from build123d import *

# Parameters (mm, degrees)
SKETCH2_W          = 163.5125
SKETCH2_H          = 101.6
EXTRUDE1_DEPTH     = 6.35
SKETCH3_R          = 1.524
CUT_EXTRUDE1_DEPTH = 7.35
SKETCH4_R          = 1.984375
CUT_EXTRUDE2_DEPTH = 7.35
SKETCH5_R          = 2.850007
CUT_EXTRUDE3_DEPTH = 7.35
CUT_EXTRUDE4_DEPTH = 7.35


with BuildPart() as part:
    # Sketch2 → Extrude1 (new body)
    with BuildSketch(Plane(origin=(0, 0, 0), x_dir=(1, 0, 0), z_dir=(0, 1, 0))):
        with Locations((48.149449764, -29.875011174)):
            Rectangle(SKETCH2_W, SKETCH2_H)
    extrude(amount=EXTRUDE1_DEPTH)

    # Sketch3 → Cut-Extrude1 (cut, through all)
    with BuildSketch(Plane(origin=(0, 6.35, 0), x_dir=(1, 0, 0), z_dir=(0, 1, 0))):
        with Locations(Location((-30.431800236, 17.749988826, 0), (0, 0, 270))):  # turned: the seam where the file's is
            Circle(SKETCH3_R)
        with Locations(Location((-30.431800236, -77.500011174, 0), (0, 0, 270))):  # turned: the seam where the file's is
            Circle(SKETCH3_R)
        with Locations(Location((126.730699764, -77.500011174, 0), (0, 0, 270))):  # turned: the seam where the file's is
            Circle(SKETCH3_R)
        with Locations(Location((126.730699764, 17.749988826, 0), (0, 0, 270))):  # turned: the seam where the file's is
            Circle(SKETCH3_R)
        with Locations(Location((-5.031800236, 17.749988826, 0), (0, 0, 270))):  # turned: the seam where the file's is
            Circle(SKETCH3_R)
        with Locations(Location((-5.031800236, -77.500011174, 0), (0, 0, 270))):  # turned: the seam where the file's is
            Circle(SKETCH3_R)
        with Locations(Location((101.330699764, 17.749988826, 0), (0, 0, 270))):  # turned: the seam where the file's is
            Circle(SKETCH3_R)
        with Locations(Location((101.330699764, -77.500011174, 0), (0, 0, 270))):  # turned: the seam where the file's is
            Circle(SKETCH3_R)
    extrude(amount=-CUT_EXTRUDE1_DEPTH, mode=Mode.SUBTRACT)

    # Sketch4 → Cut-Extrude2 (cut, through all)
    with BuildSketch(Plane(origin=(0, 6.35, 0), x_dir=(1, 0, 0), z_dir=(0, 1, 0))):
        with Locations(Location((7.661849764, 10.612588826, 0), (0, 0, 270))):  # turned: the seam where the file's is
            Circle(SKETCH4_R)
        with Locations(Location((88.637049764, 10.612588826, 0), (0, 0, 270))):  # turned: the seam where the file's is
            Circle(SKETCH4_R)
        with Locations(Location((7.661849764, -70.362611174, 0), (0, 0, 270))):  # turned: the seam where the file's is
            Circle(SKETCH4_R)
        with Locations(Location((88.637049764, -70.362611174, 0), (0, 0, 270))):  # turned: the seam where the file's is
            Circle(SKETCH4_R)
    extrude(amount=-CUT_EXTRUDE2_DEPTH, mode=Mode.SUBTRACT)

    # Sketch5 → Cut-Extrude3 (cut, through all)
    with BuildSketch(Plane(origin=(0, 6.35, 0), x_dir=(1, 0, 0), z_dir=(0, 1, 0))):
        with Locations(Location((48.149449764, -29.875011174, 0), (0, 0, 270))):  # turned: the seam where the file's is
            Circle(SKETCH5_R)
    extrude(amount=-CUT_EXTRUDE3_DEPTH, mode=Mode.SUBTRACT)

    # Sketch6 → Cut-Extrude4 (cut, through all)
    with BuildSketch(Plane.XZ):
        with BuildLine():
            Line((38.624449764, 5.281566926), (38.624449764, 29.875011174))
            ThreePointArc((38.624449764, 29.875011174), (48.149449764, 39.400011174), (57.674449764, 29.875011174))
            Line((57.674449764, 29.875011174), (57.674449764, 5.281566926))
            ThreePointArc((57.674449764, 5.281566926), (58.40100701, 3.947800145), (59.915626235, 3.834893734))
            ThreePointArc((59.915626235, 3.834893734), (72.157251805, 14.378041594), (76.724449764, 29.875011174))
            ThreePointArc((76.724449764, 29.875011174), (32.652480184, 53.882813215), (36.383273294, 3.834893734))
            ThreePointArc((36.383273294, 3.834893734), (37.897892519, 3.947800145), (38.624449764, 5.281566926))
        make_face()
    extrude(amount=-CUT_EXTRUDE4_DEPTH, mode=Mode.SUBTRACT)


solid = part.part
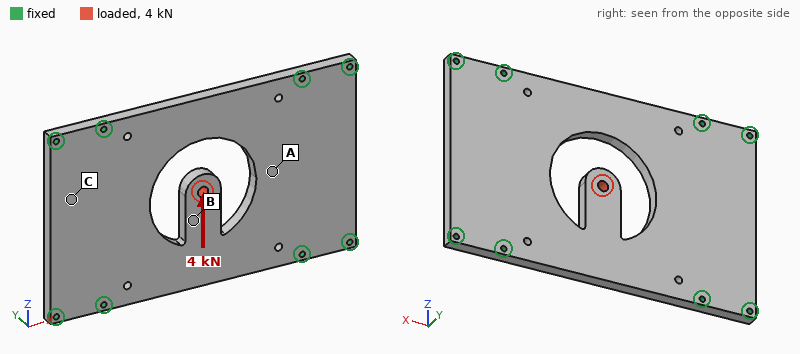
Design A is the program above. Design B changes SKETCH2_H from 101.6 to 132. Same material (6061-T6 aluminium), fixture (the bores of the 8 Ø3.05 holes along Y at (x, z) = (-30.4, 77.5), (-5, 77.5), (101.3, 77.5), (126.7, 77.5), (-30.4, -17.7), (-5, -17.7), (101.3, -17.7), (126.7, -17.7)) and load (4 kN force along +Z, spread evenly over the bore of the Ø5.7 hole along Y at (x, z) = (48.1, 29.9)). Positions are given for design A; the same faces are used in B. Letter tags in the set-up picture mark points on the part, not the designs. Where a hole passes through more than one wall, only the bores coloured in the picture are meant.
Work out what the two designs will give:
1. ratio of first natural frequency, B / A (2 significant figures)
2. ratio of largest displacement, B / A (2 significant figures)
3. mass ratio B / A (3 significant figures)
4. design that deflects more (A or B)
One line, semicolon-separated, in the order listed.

1.1; 0.82; 1.34; A
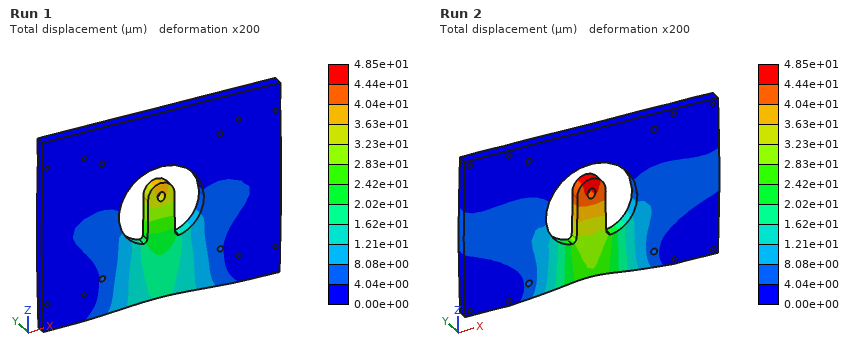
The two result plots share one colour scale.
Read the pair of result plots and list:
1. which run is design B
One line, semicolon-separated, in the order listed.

Run 1
